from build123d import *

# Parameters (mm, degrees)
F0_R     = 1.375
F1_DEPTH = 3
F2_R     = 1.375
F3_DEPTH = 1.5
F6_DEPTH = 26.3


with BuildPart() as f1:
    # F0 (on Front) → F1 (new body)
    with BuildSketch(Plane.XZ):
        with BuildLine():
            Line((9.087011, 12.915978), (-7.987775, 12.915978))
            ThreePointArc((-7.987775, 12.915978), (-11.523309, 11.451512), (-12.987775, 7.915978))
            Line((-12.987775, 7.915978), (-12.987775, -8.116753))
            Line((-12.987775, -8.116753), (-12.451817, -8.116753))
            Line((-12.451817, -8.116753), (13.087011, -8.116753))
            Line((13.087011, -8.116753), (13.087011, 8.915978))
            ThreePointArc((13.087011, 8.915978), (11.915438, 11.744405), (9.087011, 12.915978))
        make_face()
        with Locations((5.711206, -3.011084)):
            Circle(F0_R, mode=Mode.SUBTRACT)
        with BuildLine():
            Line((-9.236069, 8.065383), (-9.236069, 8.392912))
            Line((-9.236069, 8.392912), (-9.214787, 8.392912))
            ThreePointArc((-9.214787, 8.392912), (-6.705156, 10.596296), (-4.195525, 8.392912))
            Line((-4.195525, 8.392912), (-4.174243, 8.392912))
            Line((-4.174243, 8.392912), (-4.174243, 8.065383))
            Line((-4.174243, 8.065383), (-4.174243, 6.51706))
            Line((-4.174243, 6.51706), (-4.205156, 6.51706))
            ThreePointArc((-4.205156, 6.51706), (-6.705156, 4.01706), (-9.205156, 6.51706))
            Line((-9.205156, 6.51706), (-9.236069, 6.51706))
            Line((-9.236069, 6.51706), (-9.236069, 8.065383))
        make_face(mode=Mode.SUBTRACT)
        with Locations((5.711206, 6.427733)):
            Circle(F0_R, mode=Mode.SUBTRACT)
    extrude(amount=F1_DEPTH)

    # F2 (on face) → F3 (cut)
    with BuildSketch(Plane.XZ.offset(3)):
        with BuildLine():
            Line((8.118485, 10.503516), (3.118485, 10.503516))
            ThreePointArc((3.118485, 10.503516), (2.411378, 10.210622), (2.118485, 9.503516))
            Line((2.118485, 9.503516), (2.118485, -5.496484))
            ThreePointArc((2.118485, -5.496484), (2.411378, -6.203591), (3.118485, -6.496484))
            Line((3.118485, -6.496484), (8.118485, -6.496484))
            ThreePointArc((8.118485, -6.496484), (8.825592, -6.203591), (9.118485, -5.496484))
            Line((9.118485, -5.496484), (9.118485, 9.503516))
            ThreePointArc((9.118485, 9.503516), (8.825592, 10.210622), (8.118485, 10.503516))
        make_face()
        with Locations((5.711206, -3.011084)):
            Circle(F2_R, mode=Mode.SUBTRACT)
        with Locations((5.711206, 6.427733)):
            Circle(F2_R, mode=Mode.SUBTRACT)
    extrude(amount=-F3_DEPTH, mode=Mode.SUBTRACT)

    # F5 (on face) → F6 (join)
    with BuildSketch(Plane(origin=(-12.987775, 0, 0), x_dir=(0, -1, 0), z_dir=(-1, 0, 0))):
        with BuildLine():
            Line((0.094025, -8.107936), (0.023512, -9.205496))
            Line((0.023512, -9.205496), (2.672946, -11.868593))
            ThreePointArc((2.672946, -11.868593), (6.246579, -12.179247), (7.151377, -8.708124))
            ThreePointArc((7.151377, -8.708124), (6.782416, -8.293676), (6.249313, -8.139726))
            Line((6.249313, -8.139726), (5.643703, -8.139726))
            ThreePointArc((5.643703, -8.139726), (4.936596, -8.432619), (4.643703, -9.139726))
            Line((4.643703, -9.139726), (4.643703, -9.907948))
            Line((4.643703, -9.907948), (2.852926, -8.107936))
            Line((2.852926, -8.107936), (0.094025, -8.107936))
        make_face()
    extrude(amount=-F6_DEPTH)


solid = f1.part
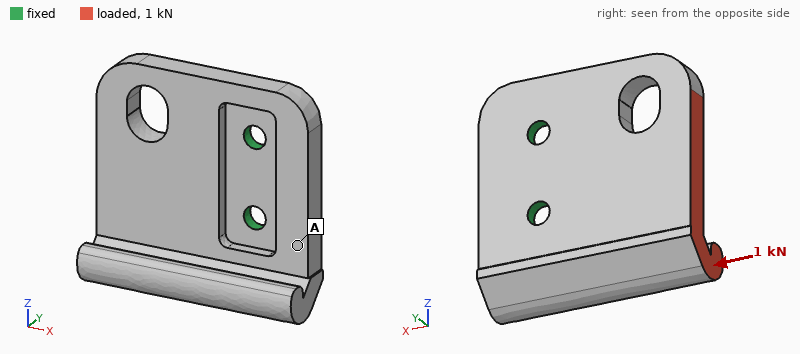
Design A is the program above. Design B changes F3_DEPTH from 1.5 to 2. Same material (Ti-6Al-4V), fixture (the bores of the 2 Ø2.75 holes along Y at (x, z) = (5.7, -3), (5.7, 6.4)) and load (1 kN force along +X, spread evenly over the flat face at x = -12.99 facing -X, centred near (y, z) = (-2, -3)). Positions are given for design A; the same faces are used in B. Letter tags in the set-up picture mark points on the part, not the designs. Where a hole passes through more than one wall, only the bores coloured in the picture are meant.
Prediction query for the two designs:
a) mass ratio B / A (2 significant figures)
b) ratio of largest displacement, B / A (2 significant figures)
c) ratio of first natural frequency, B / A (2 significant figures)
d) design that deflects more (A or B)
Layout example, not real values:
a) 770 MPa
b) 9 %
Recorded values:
a) 0.97
b) 2.2
c) 0.71
d) B
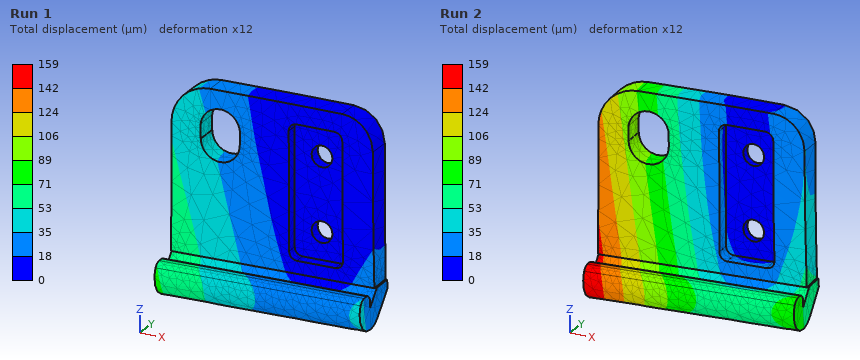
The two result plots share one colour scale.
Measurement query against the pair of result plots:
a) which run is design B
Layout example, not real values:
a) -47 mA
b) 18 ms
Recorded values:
a) Run 2
